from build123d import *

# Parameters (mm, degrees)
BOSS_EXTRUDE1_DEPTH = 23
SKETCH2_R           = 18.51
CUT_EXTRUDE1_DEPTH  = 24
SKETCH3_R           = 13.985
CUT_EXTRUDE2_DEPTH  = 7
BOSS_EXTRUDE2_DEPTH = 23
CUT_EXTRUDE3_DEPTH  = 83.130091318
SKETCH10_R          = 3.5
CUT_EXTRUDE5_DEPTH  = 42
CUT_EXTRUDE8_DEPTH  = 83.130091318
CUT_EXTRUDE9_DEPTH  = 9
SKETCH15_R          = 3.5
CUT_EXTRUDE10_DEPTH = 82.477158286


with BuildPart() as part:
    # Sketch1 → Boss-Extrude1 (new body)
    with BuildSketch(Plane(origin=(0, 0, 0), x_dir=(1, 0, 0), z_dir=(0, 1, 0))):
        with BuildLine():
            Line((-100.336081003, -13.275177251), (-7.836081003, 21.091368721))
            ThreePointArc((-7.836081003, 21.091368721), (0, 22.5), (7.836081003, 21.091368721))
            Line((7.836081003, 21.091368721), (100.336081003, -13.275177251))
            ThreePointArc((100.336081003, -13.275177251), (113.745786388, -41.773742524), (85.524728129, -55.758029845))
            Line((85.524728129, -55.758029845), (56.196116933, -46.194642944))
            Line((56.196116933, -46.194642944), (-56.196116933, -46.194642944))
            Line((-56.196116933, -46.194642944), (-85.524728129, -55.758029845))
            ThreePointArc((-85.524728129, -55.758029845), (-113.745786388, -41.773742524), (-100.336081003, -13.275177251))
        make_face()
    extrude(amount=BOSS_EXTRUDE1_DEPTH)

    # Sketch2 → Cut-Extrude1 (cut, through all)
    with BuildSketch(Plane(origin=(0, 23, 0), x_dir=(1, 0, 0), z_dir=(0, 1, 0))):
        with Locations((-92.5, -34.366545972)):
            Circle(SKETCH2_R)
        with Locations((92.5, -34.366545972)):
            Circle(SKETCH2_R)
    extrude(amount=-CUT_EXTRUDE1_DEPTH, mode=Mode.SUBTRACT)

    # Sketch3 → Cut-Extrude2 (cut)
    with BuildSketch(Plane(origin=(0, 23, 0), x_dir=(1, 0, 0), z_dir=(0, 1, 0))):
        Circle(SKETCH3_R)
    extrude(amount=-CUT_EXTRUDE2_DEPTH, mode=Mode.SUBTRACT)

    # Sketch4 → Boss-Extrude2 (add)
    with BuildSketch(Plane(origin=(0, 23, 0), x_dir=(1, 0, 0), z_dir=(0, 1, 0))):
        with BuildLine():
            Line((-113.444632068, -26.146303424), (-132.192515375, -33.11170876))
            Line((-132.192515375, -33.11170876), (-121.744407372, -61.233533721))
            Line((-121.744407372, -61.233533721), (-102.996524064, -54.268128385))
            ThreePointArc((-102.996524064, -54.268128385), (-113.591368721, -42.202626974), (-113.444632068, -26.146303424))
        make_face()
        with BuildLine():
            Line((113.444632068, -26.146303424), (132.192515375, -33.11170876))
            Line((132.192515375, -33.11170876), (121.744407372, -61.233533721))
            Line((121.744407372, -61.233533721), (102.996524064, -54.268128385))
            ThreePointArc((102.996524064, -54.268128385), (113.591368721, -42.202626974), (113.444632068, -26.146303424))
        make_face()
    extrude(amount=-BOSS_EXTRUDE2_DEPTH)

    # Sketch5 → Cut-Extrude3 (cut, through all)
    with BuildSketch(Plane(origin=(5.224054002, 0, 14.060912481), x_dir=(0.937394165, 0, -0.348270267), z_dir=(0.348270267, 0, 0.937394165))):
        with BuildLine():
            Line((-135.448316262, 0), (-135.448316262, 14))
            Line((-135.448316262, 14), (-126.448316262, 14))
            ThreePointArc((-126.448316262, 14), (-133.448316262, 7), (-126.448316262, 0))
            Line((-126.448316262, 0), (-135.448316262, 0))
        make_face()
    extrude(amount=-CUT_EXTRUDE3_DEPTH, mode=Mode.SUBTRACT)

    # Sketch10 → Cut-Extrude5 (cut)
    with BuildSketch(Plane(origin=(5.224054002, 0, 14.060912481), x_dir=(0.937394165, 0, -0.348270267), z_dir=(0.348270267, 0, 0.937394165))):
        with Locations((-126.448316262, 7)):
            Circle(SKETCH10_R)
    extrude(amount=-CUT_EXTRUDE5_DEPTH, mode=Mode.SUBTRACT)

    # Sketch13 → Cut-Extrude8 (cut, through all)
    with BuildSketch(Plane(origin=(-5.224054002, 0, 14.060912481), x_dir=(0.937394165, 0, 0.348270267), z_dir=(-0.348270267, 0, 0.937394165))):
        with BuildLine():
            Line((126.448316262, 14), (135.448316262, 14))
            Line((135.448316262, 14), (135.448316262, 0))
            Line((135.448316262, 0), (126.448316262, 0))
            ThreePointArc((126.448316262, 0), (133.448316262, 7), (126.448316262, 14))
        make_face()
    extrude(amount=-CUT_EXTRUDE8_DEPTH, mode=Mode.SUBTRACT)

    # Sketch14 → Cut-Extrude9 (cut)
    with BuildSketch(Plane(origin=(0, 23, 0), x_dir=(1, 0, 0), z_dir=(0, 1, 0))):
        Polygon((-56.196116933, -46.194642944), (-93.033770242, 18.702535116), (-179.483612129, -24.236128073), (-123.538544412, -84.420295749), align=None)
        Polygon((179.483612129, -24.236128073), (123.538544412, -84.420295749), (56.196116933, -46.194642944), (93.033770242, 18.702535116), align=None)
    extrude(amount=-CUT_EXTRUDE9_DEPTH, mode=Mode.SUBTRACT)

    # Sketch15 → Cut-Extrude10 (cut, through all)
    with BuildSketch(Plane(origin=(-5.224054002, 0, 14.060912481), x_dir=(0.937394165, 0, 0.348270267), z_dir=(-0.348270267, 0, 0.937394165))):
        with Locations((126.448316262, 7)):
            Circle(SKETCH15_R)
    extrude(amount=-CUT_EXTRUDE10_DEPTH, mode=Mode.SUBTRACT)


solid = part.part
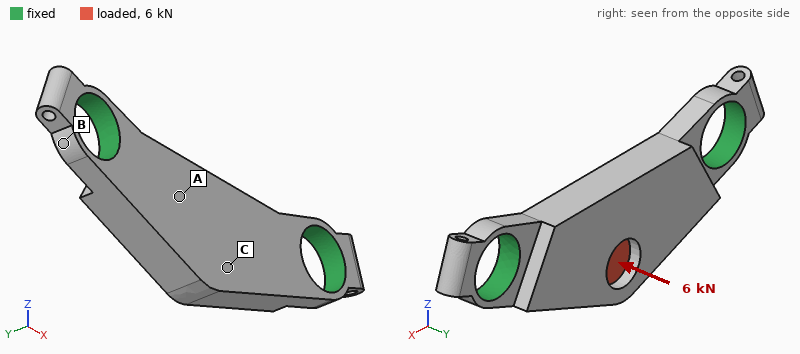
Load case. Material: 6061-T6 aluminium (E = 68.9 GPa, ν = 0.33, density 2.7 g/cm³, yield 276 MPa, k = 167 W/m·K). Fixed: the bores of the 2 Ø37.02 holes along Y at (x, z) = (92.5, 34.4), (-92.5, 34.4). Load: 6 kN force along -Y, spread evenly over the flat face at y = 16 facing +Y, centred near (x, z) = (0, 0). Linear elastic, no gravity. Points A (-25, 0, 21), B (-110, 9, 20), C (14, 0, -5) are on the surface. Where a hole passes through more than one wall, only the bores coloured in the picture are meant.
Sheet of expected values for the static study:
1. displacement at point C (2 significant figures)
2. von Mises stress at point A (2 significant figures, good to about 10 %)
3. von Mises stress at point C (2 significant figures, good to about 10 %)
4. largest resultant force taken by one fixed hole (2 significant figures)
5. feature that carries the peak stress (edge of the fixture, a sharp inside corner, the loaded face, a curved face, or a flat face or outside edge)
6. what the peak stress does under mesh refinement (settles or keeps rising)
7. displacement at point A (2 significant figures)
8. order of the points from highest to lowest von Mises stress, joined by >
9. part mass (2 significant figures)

0.12 mm
18 MPa
25 MPa
4.5 kN
edge of the fixture
keeps rising
0.063 mm
C > A > B
570 g
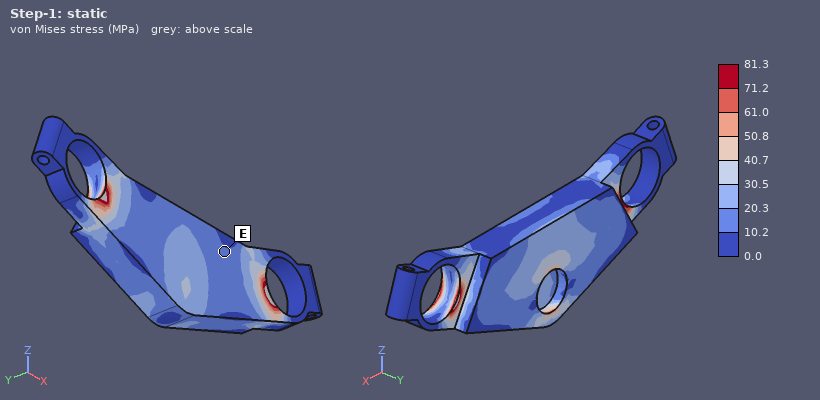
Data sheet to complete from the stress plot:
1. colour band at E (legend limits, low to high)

10.2 to 20.3 MPa
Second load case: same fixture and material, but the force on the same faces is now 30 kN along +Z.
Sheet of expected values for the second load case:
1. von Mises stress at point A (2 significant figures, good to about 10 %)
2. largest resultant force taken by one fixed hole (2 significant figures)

20 MPa
17 kN
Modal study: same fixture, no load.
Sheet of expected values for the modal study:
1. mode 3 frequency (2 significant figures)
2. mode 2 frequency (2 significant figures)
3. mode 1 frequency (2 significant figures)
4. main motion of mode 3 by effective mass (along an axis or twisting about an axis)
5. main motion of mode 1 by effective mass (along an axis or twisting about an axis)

5900 Hz
4900 Hz
2600 Hz
along Z
along Y
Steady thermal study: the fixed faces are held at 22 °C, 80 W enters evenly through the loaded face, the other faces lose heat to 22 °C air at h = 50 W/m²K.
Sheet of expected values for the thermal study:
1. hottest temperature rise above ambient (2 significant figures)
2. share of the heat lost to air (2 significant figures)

23 K
15 %
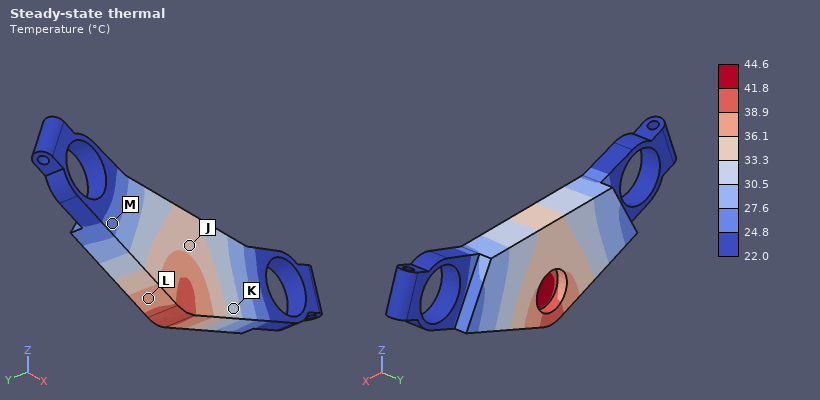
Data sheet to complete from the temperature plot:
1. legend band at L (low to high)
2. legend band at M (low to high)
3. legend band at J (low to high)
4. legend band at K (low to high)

36.1 to 38.9 °C
24.8 to 27.6 °C
33.3 to 36.1 °C
30.5 to 33.3 °C
